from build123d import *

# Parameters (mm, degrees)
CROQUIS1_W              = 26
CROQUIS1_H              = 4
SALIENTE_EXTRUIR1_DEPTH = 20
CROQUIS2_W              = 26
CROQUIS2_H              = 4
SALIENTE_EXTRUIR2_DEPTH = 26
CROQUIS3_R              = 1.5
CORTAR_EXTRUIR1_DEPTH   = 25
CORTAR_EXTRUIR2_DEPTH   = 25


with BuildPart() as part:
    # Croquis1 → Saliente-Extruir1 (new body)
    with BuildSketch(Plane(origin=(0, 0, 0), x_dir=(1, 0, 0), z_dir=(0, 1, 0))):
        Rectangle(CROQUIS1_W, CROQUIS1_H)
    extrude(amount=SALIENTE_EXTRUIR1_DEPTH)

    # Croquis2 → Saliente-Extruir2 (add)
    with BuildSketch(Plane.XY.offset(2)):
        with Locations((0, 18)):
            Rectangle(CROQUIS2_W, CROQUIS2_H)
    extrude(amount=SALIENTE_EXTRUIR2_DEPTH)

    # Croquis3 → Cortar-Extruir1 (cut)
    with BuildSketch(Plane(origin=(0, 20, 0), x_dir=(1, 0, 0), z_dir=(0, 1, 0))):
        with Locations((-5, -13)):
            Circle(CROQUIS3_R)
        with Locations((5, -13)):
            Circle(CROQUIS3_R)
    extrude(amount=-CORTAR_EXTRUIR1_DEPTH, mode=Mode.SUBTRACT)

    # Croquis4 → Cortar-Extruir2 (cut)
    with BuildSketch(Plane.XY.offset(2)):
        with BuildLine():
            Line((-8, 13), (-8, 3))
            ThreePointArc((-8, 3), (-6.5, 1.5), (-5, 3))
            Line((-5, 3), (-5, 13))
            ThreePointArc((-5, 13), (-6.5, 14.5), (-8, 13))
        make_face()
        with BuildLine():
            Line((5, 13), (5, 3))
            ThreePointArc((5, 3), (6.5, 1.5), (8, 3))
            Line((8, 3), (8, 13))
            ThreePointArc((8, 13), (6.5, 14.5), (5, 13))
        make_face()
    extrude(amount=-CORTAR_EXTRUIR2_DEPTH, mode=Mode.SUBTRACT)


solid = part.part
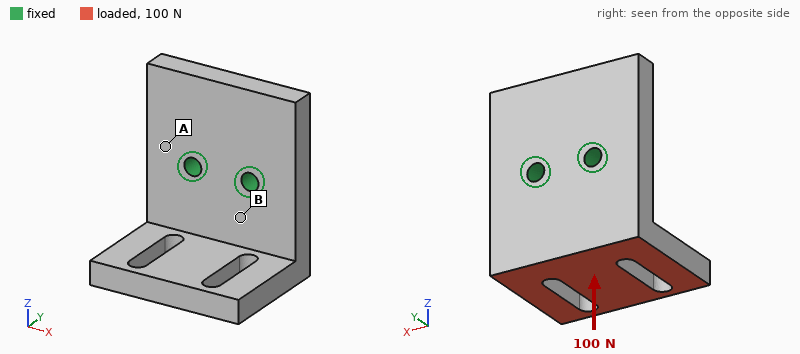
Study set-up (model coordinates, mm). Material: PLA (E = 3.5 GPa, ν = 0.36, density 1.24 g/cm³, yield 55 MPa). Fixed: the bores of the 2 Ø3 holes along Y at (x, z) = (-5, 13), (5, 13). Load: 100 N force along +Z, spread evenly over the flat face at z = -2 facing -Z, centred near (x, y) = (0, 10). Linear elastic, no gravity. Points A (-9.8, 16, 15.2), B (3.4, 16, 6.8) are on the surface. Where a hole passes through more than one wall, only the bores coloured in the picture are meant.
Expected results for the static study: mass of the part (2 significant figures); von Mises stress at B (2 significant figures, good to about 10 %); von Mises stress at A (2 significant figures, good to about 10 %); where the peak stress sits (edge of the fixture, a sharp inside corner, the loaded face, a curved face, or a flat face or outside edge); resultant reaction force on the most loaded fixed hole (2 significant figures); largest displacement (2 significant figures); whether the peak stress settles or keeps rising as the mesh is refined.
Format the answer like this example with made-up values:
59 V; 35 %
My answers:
5.5 g; 12 MPa; 2.5 MPa; edge of the fixture; 51 N; 0.50 mm; keeps rising
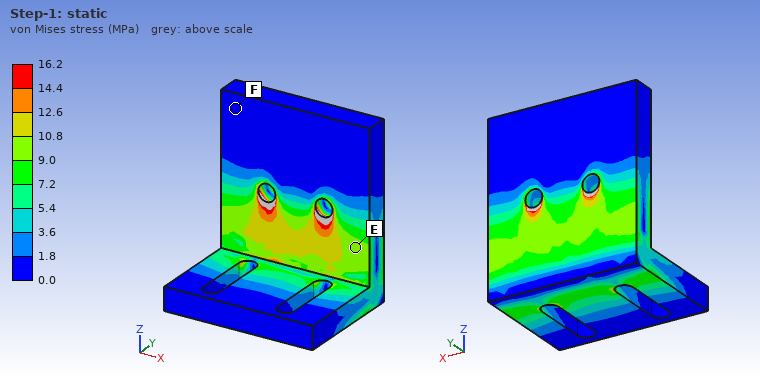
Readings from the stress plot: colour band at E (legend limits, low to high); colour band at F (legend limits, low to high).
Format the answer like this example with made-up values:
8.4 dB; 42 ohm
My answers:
9.0 to 10.8 MPa; 0.0 to 1.8 MPa
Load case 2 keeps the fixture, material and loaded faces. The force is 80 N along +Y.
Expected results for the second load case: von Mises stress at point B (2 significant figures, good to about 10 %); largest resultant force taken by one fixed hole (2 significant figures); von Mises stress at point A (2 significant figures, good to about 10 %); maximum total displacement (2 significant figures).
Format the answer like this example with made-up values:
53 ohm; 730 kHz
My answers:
9.7 MPa; 40 N; 3.2 MPa; 0.40 mm
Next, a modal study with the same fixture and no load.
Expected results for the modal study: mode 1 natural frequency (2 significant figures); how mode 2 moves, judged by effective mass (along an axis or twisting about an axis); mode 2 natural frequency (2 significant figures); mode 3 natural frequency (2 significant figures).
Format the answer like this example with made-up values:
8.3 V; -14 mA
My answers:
1600 Hz; along X; 2500 Hz; 4100 Hz
